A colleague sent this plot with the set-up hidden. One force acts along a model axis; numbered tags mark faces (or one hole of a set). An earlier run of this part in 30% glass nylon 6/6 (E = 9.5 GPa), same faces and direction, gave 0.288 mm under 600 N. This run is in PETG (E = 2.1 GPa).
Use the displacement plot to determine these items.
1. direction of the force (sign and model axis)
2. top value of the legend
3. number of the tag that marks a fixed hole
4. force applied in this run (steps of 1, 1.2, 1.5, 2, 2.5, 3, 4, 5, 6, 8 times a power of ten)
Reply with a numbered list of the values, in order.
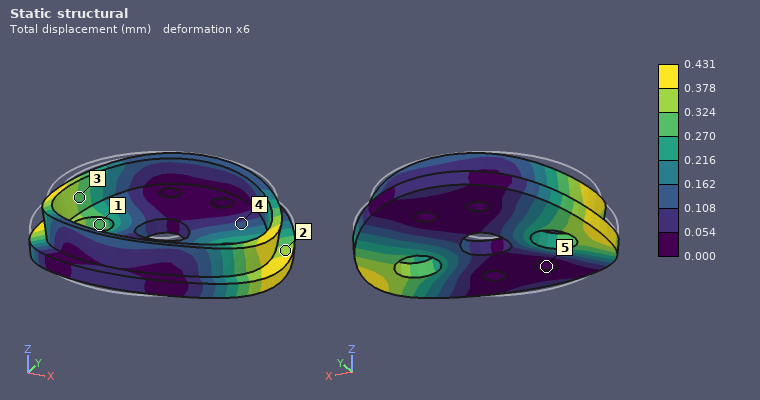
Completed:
1. -Z
2. 0.431 mm
3. 5
4. 200 N
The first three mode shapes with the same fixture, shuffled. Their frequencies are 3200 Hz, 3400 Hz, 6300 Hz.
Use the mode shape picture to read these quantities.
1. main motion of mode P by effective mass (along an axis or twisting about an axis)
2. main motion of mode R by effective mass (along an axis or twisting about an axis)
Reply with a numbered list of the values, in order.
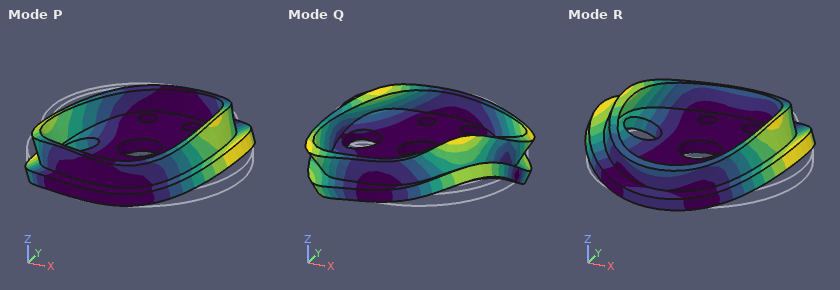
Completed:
1. twisting about Y
2. along Z
